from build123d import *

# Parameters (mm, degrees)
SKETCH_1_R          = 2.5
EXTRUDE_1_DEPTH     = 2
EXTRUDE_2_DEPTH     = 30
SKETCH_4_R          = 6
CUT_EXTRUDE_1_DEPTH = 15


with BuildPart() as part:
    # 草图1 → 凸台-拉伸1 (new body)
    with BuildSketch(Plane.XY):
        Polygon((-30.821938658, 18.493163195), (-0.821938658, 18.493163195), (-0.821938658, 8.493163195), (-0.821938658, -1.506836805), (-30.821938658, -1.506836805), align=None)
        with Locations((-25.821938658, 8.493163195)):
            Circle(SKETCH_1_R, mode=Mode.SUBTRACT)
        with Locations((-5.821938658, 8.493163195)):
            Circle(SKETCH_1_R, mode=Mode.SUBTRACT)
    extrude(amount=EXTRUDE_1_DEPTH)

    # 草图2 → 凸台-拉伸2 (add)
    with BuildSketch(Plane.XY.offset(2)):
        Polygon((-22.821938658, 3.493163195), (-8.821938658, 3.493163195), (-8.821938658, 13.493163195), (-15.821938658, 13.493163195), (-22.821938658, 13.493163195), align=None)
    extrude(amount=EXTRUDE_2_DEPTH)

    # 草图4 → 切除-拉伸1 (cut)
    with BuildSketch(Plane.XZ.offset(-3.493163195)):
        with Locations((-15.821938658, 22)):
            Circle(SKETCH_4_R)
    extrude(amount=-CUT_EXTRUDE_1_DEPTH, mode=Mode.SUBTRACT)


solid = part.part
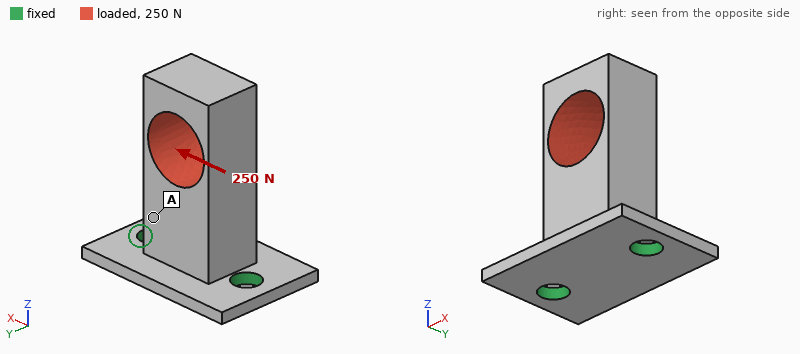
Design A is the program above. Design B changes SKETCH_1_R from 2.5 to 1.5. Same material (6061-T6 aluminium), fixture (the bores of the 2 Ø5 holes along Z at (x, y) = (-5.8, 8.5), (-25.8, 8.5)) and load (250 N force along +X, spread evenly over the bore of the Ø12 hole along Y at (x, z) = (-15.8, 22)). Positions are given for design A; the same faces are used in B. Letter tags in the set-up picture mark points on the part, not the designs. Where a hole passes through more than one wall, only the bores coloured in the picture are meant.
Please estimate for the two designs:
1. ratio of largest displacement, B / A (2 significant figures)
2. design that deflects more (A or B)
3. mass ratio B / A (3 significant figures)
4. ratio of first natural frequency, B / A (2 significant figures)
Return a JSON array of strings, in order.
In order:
["1.2", "B", "1.01", "0.74"]
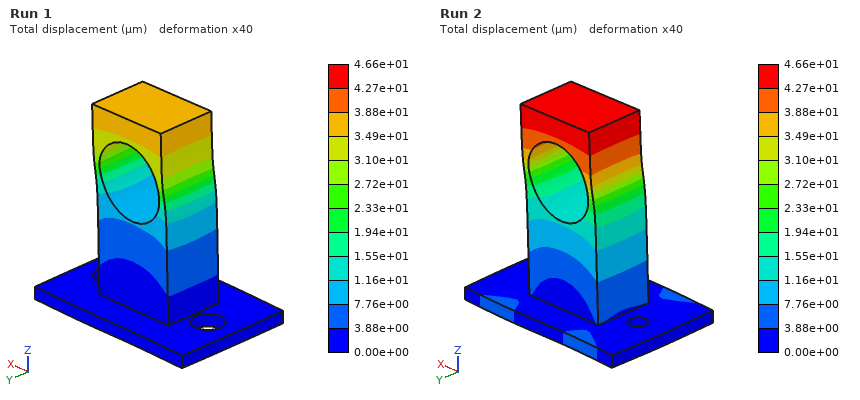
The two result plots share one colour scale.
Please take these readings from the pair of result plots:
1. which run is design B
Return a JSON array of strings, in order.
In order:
["Run 2"]
